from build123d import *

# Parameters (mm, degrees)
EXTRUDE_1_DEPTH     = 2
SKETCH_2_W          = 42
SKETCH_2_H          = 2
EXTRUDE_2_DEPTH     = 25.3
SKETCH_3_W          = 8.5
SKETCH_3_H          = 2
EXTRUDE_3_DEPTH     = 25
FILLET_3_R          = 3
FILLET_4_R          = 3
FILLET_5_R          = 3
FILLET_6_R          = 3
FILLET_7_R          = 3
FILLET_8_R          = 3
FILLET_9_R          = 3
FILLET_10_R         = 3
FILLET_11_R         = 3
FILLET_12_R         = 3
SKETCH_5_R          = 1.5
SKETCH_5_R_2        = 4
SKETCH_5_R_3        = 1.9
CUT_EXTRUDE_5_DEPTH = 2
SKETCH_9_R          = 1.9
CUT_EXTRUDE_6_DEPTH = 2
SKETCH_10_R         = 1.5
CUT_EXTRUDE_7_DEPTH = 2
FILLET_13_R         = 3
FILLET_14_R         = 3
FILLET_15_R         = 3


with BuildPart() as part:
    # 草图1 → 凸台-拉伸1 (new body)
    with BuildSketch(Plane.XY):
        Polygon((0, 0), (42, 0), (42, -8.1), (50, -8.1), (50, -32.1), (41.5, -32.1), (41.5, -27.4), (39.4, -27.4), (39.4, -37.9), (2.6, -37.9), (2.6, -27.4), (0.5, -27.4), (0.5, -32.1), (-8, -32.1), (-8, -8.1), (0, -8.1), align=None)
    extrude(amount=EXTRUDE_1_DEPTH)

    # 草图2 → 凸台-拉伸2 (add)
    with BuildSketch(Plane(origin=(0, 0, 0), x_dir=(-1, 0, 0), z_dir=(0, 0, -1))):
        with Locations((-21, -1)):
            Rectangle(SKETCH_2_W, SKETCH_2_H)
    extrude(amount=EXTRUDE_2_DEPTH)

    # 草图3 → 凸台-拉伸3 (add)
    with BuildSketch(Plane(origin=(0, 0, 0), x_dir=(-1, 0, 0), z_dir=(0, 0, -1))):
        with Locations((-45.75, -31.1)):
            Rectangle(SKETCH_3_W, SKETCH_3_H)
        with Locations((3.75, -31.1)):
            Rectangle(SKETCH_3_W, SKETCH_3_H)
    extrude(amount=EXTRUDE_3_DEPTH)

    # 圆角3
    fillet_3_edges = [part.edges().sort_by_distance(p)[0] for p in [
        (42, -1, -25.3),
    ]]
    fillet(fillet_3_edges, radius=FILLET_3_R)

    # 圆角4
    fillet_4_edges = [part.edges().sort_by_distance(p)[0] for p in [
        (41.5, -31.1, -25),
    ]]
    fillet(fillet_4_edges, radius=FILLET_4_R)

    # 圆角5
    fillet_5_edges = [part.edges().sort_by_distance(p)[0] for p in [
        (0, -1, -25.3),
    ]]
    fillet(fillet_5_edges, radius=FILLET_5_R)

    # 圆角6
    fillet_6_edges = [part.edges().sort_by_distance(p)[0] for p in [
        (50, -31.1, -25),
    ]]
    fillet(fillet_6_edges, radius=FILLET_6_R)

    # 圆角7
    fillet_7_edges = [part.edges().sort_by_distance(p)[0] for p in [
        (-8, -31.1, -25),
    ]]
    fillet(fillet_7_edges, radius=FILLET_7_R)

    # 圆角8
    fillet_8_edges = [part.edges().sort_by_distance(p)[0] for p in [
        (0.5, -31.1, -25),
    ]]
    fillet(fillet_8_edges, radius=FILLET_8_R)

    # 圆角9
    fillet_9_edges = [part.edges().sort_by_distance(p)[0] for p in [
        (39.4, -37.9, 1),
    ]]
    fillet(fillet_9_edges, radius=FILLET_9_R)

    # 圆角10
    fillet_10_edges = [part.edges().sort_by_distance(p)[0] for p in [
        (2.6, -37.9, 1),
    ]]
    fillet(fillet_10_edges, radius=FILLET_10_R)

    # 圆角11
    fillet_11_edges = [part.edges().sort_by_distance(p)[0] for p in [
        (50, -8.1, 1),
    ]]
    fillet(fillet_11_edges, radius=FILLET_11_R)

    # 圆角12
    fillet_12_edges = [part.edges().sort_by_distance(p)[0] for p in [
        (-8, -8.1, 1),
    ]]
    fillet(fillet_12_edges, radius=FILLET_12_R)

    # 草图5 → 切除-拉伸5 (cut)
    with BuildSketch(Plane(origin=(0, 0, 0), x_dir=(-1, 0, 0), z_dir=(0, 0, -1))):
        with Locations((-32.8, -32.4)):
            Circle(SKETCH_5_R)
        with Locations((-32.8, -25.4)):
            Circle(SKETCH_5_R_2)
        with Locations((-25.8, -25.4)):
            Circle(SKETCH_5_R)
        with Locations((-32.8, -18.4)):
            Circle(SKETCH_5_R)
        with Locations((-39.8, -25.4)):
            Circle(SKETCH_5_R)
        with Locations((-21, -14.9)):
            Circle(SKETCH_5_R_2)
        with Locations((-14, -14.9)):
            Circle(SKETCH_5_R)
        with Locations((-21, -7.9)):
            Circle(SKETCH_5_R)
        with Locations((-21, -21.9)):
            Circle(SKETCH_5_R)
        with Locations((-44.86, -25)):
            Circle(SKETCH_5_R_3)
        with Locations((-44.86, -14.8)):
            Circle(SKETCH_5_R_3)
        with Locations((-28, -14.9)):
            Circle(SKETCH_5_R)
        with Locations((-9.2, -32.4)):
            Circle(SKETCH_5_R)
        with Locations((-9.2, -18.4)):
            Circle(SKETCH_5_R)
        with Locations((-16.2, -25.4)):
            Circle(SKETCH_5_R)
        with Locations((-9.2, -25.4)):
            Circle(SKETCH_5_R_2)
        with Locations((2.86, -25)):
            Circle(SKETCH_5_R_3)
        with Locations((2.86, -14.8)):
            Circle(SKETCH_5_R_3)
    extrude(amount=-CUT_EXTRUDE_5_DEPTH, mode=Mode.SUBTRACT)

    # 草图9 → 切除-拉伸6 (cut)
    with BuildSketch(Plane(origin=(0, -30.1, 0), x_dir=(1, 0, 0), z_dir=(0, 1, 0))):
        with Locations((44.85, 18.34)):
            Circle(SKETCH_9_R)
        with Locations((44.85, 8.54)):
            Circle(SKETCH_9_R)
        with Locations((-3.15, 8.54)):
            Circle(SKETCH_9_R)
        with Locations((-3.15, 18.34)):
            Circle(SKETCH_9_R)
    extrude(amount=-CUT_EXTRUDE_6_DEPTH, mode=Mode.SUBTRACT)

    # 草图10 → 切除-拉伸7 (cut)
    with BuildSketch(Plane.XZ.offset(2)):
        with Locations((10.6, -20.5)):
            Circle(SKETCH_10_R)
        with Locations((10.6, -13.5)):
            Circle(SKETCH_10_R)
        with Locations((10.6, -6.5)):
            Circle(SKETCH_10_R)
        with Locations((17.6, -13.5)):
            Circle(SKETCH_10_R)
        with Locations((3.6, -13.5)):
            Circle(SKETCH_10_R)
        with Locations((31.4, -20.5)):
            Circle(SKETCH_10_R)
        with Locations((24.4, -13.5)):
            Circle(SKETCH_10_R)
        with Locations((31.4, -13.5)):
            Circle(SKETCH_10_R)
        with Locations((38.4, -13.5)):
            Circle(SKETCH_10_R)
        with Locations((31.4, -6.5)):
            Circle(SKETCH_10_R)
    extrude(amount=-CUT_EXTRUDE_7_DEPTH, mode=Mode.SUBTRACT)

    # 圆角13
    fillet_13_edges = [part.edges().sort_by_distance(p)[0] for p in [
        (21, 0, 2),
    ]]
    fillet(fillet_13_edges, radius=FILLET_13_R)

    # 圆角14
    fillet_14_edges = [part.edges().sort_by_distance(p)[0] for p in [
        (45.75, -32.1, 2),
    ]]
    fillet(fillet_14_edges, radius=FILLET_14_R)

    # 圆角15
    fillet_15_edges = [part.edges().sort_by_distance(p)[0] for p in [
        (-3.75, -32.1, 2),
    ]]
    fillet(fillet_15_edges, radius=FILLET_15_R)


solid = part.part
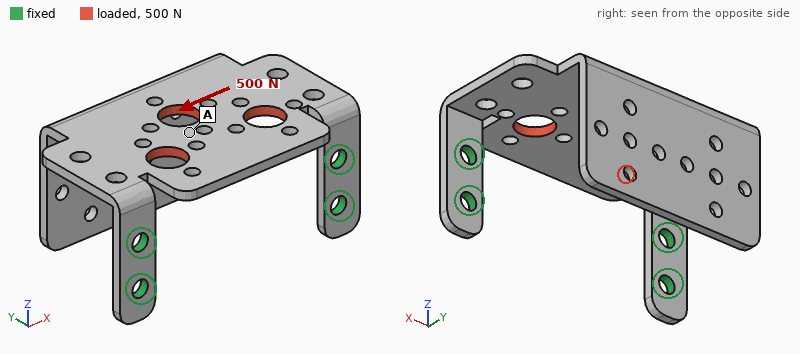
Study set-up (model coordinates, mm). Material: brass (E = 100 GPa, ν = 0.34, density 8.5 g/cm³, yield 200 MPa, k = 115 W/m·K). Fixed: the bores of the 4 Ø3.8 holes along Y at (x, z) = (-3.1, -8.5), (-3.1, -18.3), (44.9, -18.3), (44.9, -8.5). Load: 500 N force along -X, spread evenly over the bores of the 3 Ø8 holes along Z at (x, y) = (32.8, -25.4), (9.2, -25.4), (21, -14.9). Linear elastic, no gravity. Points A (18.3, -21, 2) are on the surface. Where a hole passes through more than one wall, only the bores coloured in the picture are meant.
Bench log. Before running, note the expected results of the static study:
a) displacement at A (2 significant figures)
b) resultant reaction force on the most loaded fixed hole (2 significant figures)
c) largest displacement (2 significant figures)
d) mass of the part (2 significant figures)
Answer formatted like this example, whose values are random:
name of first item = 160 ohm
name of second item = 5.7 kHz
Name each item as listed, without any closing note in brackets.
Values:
displacement at A = 32 µm
resultant reaction force on the most loaded fixed hole = 340 N
largest displacement = 96 µm
mass of the part = 50 g
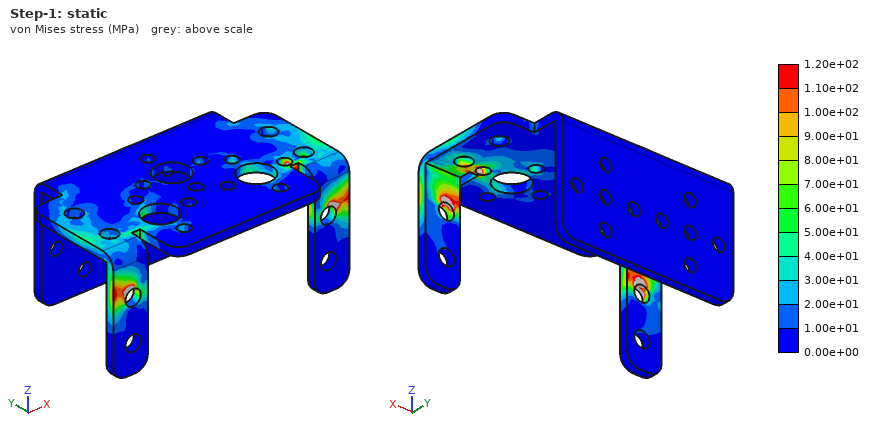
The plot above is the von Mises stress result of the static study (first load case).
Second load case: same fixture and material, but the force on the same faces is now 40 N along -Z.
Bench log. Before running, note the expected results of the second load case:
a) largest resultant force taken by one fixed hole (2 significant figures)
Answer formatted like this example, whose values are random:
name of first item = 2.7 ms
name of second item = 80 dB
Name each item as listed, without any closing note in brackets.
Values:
largest resultant force taken by one fixed hole = 21 N
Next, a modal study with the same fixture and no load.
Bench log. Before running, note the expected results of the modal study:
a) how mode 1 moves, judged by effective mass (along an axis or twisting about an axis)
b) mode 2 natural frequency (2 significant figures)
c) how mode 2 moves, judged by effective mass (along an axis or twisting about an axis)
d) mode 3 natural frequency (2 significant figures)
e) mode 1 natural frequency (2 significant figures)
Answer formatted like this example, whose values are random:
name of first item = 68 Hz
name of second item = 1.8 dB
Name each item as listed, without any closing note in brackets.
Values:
how mode 1 moves, judged by effective mass = along Z
mode 2 natural frequency = 730 Hz
how mode 2 moves, judged by effective mass = along X
mode 3 natural frequency = 960 Hz
mode 1 natural frequency = 250 Hz
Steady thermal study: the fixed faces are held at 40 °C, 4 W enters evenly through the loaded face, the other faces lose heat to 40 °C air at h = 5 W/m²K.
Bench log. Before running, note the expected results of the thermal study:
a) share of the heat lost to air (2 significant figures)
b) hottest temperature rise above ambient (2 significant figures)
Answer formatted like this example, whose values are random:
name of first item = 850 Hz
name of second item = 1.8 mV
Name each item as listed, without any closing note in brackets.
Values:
share of the heat lost to air = 15 %
hottest temperature rise above ambient = 23 K
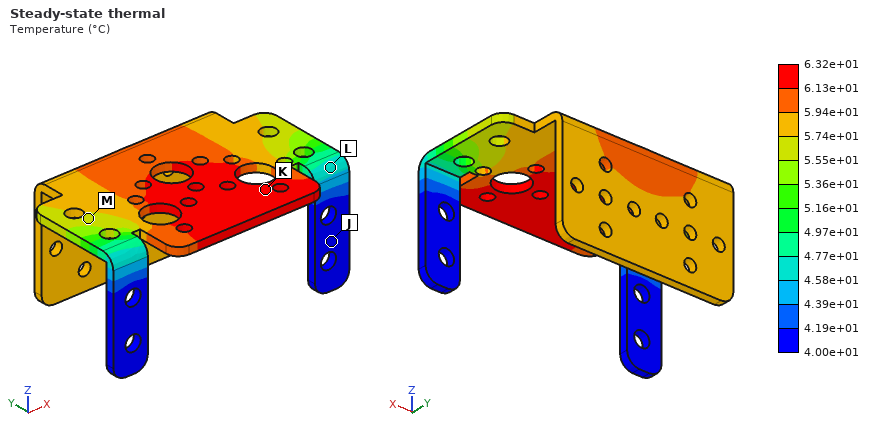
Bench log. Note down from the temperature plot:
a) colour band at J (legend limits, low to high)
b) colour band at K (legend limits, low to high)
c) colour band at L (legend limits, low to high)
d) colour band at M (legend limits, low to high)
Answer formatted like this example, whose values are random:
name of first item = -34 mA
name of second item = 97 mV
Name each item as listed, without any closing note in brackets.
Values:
colour band at J = 4.00e+01 to 4.19e+01 °C
colour band at K = 6.13e+01 to 6.32e+01 °C
colour band at L = 4.58e+01 to 4.77e+01 °C
colour band at M = 5.55e+01 to 5.74e+01 °C
